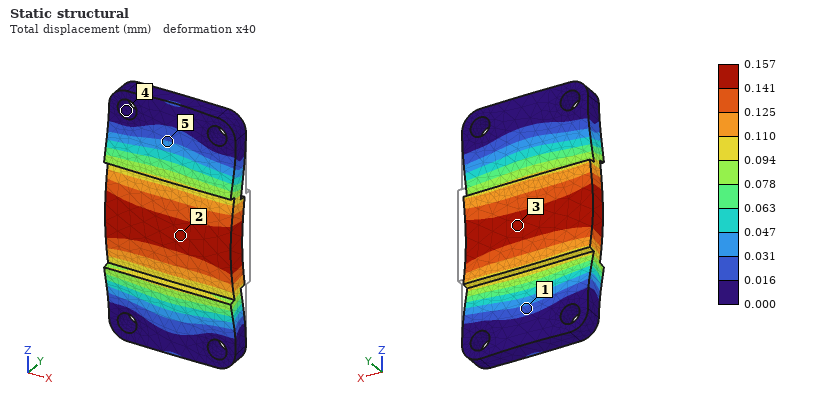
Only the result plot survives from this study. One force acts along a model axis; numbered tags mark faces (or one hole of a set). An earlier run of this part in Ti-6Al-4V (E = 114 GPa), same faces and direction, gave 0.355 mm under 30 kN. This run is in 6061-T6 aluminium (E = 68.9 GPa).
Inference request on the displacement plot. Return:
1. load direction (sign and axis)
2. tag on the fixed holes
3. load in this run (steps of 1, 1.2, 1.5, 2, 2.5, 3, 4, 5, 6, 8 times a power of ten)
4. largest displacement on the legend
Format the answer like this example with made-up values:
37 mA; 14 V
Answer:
-Y; 4; 8 kN; 0.157 mm
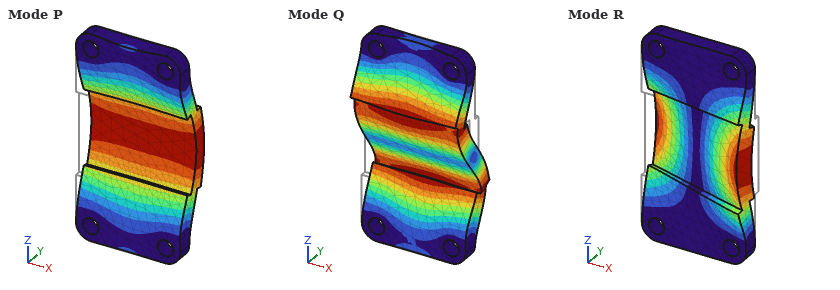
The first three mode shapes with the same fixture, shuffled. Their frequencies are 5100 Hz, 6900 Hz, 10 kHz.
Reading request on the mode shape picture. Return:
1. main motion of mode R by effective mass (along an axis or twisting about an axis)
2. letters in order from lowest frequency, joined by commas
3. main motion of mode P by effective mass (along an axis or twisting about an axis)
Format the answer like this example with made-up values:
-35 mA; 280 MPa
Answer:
twisting about Z; P, R, Q; along Y
